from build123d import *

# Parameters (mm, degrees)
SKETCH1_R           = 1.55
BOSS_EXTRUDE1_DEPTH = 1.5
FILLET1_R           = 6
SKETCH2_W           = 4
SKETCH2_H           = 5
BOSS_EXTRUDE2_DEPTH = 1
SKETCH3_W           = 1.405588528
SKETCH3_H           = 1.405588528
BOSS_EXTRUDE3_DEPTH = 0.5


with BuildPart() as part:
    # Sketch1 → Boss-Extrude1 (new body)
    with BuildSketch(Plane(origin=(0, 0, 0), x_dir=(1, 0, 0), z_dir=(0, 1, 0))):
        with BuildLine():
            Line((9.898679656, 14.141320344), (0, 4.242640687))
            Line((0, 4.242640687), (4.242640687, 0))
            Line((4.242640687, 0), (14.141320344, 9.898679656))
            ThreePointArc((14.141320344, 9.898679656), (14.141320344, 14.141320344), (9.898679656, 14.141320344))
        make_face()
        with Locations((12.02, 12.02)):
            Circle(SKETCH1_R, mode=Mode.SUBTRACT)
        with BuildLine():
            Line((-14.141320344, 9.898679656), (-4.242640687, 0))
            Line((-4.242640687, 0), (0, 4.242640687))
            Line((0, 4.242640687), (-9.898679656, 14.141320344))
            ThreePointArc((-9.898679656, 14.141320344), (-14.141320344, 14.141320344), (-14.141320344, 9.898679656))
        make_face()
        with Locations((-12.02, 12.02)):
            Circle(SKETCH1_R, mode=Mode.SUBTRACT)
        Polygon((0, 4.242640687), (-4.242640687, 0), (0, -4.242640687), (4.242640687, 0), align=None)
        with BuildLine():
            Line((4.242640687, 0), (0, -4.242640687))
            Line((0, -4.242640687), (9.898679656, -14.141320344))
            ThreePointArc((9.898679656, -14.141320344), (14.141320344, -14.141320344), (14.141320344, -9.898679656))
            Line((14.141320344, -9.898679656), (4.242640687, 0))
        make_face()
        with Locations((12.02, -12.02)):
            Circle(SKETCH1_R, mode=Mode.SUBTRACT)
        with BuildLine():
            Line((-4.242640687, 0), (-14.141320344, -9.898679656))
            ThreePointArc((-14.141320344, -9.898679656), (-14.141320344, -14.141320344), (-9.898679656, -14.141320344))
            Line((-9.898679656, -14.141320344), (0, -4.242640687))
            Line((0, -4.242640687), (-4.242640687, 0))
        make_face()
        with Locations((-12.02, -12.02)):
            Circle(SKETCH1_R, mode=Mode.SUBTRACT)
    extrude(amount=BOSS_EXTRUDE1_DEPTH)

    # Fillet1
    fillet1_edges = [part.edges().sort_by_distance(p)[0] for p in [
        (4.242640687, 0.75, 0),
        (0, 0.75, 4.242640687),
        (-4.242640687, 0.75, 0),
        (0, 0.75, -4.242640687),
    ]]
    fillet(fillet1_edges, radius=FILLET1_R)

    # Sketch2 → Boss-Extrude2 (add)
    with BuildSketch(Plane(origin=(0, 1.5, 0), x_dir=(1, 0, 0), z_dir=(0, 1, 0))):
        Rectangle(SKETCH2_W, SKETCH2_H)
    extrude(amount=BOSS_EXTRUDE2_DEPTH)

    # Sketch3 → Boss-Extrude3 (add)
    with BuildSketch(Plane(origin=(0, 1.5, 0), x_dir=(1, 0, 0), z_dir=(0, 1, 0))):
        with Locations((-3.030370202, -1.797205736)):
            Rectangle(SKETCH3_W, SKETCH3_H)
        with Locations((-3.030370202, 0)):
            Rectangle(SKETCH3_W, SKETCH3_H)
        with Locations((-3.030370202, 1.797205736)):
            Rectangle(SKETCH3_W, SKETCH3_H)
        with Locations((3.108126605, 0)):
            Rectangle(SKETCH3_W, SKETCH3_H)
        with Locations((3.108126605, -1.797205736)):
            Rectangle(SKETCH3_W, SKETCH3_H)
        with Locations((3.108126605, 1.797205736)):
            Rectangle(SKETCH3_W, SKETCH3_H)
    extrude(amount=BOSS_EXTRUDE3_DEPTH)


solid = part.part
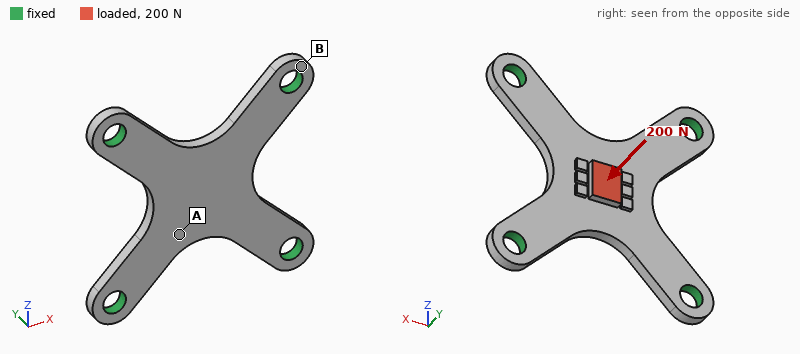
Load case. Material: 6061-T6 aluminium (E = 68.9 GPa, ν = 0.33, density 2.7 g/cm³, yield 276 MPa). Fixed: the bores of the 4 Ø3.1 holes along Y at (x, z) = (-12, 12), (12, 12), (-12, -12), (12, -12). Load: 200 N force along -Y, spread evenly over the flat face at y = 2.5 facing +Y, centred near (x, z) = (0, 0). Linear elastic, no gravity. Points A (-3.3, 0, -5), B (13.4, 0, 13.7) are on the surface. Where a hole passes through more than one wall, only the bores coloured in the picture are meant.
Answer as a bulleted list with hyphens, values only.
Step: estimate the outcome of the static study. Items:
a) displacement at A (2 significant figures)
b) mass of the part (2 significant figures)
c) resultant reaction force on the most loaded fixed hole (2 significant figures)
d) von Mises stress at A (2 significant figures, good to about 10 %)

- 64 µm
- 1.8 g
- 51 N
- 55 MPa
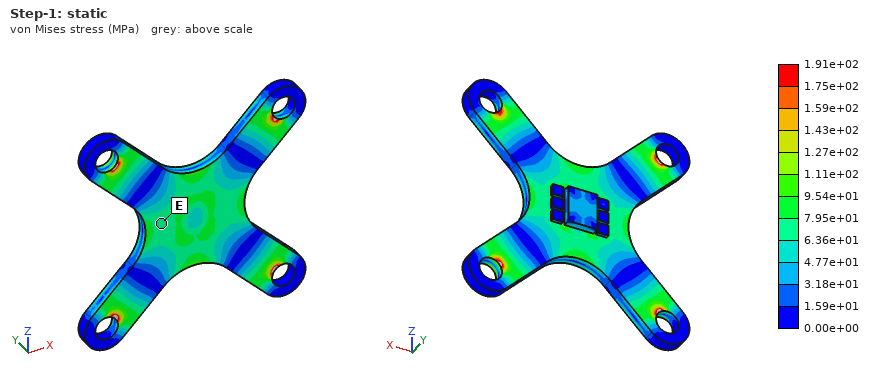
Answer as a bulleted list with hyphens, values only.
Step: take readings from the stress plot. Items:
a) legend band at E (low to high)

- 6.36e+01 to 7.95e+01 MPa
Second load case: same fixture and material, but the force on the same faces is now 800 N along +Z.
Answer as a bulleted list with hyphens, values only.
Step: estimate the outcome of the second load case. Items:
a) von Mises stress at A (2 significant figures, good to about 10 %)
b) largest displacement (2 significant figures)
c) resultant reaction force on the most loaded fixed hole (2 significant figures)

- 43 MPa
- 45 µm
- 260 N
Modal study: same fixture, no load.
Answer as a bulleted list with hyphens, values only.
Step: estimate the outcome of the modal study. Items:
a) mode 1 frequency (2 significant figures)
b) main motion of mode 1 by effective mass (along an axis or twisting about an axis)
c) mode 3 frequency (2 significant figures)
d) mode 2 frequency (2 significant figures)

- 9400 Hz
- along Y
- 21 kHz
- 21 kHz
